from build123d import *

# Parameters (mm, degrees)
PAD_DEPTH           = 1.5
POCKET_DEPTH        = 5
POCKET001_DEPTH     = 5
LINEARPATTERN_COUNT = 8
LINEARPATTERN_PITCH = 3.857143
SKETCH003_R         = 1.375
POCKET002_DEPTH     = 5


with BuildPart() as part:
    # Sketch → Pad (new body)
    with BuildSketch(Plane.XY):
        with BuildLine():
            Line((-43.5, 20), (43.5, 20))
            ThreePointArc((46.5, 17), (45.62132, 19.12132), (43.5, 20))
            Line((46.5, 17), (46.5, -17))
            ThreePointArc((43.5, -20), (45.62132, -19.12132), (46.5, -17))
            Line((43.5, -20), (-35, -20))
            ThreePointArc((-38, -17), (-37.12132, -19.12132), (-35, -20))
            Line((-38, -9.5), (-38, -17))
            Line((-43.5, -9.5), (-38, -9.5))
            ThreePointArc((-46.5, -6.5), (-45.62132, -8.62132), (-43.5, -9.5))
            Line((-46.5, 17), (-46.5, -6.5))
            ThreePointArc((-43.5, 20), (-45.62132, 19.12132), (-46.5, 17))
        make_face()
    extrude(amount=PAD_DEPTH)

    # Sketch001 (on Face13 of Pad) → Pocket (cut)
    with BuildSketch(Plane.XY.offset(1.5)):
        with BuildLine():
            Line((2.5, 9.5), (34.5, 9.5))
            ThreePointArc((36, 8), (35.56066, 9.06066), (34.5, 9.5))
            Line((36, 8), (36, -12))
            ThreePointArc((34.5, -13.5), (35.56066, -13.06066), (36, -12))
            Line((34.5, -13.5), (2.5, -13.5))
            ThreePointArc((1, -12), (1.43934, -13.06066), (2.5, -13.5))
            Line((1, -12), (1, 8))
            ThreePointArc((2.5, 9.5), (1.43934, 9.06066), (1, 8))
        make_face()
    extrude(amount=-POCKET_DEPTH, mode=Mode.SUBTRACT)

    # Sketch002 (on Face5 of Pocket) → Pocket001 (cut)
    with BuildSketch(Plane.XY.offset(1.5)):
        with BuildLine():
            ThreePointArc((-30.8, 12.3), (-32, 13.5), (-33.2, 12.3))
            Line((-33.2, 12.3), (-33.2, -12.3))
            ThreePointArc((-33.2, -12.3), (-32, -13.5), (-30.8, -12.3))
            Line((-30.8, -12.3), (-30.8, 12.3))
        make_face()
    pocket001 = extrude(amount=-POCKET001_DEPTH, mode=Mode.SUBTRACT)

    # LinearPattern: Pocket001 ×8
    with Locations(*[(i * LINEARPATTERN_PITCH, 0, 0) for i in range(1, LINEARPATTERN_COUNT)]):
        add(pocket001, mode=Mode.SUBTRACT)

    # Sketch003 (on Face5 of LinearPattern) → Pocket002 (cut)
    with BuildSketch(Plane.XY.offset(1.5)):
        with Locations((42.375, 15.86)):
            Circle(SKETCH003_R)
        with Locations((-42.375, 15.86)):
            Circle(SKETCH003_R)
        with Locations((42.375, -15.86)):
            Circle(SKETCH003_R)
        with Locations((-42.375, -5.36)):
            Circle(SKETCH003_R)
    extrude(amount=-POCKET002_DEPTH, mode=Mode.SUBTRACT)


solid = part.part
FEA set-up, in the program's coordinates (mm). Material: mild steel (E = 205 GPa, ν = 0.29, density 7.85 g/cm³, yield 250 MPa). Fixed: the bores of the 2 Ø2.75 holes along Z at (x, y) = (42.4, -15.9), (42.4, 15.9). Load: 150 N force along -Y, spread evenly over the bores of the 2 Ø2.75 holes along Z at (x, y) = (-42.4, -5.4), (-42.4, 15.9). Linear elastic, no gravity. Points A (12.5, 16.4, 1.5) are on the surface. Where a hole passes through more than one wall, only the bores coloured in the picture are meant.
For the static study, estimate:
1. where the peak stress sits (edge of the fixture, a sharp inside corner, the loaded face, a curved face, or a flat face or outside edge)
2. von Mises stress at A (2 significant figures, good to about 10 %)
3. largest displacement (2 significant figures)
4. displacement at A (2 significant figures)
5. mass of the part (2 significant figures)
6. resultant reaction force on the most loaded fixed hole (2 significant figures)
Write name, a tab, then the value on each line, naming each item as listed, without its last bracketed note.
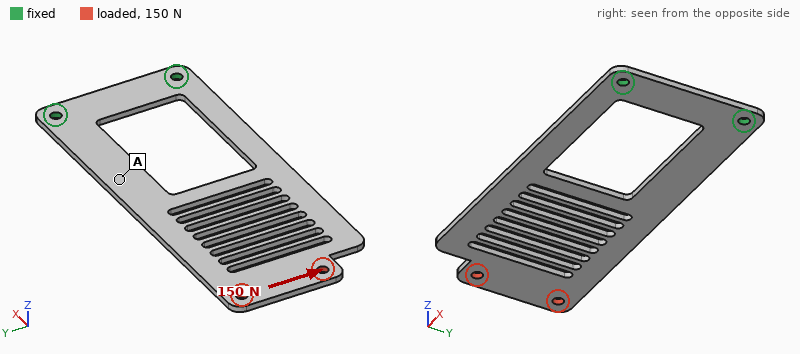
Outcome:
where the peak stress sits	a curved face
von Mises stress at A	27 MPa
largest displacement	0.16 mm
displacement at A	0.044 mm
mass of the part	27 g
resultant reaction force on the most loaded fixed hole	370 N
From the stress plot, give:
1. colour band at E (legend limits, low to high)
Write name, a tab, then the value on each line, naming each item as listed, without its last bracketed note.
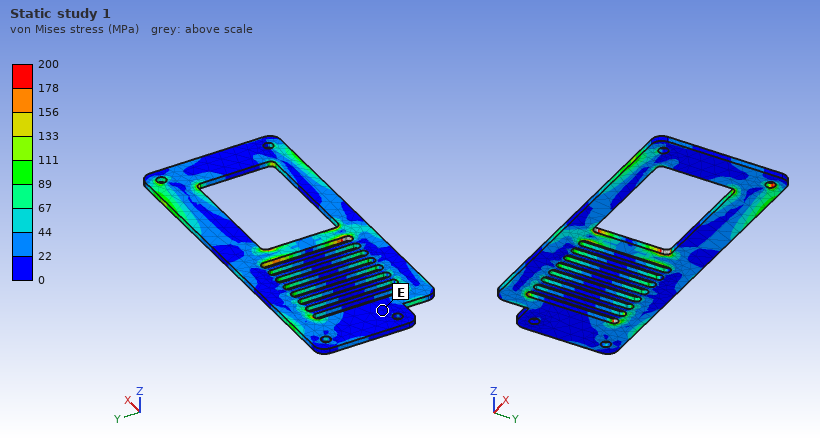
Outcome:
colour band at E	0 to 22 MPa
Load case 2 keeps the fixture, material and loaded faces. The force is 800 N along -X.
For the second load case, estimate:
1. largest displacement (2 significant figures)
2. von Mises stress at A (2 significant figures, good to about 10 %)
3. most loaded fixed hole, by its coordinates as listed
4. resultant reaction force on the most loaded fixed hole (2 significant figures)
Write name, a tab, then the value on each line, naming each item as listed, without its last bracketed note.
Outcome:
largest displacement	33 µm
von Mises stress at A	39 MPa
most loaded fixed hole, by its coordinates as listed	(42.4, 15.9)
resultant reaction force on the most loaded fixed hole	530 N
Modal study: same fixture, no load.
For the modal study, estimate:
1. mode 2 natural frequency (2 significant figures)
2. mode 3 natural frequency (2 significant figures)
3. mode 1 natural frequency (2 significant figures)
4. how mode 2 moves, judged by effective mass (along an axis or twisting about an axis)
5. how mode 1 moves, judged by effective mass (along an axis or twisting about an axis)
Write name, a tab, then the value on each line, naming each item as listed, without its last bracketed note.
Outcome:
mode 2 natural frequency	590 Hz
mode 3 natural frequency	810 Hz
mode 1 natural frequency	130 Hz
how mode 2 moves, judged by effective mass	twisting about X
how mode 1 moves, judged by effective mass	along Z
